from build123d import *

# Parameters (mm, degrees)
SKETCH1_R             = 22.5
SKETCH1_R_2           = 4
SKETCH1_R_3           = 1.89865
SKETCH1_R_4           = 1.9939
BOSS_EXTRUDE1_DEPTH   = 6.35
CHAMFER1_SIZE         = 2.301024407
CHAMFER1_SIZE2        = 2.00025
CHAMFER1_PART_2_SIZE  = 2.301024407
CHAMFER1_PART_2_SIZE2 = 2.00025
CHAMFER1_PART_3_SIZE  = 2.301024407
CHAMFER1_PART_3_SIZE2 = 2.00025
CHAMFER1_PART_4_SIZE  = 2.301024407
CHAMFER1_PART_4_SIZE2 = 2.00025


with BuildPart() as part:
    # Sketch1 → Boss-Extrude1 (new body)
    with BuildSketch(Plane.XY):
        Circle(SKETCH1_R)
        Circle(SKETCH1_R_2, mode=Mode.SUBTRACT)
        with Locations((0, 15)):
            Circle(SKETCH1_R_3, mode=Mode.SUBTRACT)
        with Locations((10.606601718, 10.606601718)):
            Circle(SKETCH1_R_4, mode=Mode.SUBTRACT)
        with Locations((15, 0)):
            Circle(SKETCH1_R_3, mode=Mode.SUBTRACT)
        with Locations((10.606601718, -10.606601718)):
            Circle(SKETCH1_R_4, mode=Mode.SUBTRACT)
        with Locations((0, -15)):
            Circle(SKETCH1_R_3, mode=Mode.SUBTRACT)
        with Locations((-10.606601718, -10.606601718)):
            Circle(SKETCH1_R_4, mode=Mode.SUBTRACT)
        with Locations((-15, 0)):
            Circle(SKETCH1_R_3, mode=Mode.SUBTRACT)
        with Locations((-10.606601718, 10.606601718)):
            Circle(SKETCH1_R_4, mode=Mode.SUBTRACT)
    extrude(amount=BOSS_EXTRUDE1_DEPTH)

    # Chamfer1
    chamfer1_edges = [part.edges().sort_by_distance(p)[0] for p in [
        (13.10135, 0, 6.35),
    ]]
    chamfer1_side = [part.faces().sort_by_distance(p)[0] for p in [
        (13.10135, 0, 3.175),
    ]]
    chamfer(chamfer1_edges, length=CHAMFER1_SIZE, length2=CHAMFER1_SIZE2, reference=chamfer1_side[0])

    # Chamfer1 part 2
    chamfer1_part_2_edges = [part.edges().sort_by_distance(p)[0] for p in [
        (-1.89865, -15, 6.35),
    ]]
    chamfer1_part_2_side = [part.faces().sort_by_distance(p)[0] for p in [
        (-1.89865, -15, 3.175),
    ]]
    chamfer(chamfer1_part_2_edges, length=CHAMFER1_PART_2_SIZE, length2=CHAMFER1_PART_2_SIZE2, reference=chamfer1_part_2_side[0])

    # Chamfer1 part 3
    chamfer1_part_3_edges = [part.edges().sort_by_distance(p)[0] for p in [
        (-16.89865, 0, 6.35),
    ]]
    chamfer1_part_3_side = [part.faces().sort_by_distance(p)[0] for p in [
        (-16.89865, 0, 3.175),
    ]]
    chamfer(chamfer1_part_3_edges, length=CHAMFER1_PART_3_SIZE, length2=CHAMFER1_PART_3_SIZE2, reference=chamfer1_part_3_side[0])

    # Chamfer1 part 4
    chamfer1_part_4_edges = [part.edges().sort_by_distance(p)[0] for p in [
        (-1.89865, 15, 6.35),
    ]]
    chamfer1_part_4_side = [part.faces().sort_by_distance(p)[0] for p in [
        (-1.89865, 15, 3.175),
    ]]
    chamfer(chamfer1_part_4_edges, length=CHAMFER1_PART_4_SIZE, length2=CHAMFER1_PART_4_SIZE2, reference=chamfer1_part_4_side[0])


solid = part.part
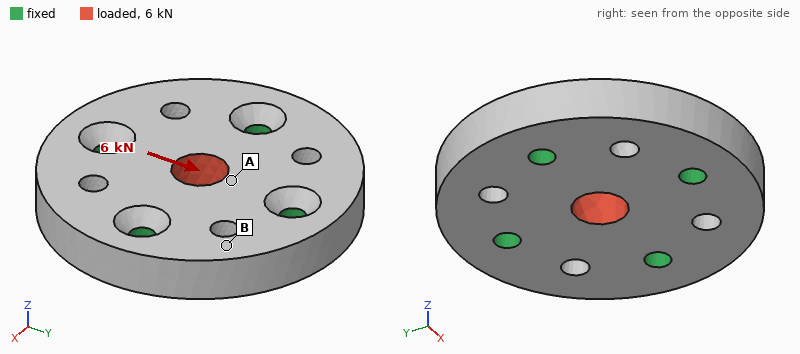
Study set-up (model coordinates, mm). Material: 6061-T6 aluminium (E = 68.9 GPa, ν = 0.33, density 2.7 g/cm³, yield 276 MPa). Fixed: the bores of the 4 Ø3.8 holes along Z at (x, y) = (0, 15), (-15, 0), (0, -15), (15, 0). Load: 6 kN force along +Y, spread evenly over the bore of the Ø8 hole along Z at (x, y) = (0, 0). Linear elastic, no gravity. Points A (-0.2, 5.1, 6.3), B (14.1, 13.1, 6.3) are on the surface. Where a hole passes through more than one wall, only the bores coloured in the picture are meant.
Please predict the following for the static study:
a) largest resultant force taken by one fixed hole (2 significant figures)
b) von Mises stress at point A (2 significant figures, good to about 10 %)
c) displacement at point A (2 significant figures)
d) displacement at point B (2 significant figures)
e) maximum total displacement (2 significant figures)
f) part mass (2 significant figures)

2.0 kN
42 MPa
5.8 µm
2.4 µm
6.8 µm
24 g
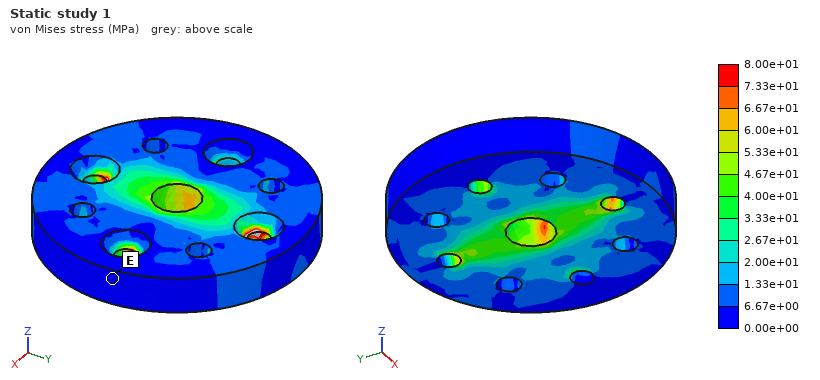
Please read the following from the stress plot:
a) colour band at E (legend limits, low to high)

0.00e+00 to 6.67e+00 MPa
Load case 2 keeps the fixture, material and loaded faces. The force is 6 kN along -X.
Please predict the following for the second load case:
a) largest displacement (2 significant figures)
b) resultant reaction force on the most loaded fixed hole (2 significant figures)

6.7 µm
2.0 kN
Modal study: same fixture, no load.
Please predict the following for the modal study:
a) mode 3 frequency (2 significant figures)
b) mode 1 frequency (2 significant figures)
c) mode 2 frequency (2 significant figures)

27 kHz
24 kHz
27 kHz
